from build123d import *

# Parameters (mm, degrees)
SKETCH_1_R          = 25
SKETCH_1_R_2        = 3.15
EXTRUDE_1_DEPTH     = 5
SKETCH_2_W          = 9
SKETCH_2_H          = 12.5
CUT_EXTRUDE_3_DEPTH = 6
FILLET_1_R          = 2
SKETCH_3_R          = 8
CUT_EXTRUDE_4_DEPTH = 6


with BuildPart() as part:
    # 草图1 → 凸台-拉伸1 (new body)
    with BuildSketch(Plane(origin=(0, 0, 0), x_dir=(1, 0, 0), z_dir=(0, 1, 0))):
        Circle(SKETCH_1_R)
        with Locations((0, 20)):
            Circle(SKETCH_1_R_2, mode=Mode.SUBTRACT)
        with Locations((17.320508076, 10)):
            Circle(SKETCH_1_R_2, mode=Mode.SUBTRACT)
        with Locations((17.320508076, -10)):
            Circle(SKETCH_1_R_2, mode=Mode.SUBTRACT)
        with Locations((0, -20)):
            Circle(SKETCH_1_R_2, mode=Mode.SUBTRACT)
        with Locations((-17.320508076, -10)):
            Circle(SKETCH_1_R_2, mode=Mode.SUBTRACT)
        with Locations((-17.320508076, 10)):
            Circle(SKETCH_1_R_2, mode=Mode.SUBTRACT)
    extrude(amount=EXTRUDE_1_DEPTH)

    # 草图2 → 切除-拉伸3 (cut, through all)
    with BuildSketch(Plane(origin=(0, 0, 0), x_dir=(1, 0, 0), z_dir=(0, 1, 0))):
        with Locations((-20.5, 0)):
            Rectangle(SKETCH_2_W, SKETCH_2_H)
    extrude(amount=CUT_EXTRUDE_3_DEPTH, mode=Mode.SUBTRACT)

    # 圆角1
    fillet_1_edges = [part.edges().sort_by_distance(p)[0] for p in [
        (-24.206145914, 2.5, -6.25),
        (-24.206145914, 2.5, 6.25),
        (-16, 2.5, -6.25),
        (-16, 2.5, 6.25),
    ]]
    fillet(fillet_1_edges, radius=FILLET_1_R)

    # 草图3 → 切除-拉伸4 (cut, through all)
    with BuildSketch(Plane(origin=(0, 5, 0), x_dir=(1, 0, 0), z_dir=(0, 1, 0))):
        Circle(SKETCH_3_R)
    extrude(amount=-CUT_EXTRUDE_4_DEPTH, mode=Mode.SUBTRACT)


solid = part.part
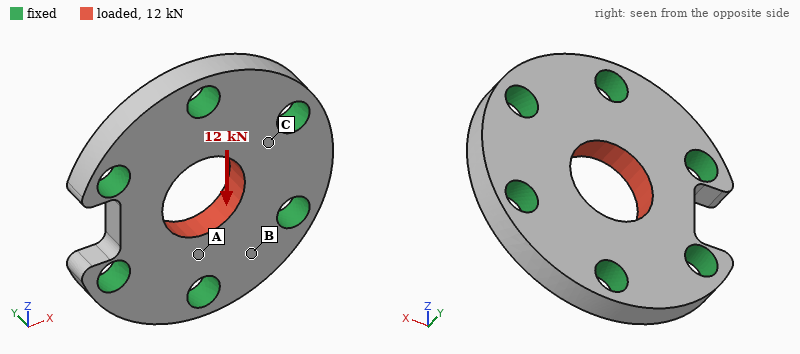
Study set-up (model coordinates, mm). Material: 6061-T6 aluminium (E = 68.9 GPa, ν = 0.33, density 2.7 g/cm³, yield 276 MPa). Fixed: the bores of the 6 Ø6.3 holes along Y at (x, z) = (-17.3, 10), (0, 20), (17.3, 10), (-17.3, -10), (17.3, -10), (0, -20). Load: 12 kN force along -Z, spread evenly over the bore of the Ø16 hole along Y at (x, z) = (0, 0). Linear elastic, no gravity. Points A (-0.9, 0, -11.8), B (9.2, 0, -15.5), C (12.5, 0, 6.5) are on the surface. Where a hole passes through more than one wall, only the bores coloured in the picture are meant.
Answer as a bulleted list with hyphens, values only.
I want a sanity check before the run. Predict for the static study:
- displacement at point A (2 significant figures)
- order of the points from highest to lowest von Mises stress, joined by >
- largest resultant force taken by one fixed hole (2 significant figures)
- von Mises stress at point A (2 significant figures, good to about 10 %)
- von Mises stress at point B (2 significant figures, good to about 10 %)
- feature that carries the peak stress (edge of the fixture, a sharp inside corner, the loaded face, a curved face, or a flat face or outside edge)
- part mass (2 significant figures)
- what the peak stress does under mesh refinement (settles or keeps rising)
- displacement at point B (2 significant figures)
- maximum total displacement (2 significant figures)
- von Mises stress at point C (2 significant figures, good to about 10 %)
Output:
- 4.7 µm
- A > C > B
- 3.1 kN
- 56 MPa
- 12 MPa
- edge of the fixture
- 20 g
- keeps rising
- 3.4 µm
- 8.5 µm
- 36 MPa
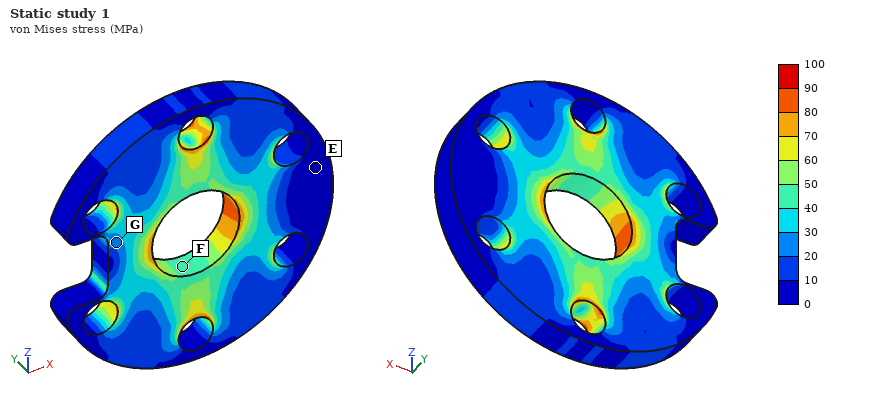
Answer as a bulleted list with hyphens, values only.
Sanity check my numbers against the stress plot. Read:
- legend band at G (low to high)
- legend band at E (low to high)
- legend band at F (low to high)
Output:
- 20 to 30 MPa
- 0 to 10 MPa
- 40 to 50 MPa
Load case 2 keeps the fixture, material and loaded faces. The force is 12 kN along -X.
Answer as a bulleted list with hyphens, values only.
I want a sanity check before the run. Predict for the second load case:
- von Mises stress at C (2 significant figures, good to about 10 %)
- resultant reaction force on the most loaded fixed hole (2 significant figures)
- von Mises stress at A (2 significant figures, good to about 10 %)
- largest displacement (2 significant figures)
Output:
- 55 MPa
- 2.7 kN
- 30 MPa
- 11 µm
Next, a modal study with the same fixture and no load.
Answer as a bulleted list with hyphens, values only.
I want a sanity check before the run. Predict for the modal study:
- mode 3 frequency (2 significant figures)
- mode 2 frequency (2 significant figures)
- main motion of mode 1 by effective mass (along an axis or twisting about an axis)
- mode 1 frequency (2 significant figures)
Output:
- 49 kHz
- 49 kHz
- along Y
- 39 kHz
